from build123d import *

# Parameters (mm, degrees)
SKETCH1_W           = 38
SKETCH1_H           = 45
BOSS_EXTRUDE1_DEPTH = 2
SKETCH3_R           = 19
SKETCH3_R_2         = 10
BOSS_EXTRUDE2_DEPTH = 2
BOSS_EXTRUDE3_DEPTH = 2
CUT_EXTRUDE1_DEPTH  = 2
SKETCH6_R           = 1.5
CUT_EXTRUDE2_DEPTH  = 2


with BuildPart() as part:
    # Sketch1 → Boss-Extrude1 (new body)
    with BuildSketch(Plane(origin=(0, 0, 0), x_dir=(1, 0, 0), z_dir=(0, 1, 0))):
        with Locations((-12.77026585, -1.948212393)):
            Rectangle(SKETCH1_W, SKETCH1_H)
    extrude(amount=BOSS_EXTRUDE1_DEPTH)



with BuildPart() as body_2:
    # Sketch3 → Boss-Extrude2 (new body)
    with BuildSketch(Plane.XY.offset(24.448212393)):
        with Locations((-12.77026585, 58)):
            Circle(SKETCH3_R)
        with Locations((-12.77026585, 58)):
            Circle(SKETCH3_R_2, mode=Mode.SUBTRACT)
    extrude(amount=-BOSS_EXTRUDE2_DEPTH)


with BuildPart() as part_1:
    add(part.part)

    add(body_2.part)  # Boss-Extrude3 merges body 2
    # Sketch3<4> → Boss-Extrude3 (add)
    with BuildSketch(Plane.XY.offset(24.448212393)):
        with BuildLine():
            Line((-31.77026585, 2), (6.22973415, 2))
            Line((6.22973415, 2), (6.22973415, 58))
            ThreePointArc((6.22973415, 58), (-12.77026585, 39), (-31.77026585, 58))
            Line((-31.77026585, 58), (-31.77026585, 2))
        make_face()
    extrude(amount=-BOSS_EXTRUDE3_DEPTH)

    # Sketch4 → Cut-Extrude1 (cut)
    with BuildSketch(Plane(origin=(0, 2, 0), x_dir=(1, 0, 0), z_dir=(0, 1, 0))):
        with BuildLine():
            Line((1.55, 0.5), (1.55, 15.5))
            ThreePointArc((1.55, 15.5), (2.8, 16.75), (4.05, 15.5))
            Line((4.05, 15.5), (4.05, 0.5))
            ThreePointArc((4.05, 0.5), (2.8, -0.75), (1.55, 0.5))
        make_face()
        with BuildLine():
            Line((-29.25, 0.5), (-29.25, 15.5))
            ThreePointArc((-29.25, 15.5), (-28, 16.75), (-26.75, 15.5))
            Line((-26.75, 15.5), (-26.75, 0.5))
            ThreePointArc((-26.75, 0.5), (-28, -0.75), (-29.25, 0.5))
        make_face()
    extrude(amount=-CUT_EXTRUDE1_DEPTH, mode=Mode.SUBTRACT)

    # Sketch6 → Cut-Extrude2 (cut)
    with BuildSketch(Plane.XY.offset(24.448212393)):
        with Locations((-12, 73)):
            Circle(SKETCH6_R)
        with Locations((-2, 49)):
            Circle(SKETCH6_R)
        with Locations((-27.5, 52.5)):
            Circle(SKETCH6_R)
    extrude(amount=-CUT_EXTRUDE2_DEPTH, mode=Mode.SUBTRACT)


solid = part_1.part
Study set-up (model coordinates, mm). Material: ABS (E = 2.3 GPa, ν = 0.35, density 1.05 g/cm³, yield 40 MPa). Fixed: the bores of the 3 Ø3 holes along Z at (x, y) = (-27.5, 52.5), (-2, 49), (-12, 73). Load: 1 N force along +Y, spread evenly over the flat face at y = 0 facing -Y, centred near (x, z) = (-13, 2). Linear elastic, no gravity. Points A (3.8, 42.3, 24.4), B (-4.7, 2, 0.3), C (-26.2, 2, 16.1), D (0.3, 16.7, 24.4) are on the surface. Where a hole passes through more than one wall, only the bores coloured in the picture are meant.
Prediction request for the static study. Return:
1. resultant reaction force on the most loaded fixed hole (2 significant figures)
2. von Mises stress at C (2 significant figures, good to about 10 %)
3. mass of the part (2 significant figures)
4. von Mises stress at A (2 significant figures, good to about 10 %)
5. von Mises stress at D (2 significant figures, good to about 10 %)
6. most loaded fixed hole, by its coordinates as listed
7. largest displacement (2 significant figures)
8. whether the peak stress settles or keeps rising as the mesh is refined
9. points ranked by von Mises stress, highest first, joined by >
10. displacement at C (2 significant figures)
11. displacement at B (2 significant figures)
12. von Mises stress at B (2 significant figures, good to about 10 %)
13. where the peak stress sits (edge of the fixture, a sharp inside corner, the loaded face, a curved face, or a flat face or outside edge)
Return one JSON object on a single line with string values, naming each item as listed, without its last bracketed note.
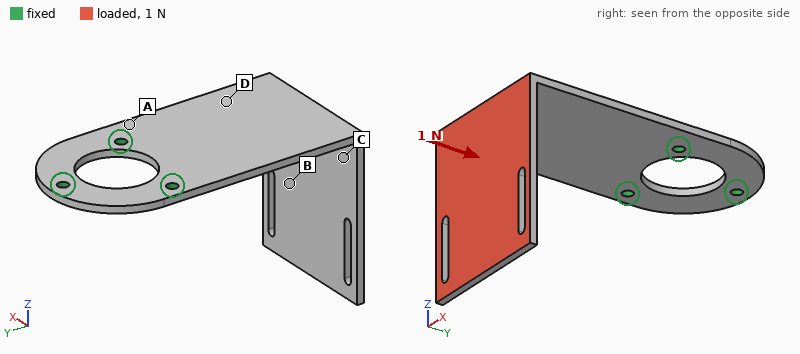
{"resultant reaction force on the most loaded fixed hole": "0.56 N", "von Mises stress at C": "0.50 MPa", "mass of the part": "8.4 g", "von Mises stress at A": "1.00 MPa", "von Mises stress at D": "0.80 MPa", "most loaded fixed hole, by its coordinates as listed": "(-2, 49)", "largest displacement": "1.0 mm", "whether the peak stress settles or keeps rising as the mesh is refined": "keeps rising", "points ranked by von Mises stress, highest first, joined by >": "A > D > C > B", "displacement at C": "0.46 mm", "displacement at B": "0.63 mm", "von Mises stress at B": "0.19 MPa", "where the peak stress sits": "edge of the fixture"}
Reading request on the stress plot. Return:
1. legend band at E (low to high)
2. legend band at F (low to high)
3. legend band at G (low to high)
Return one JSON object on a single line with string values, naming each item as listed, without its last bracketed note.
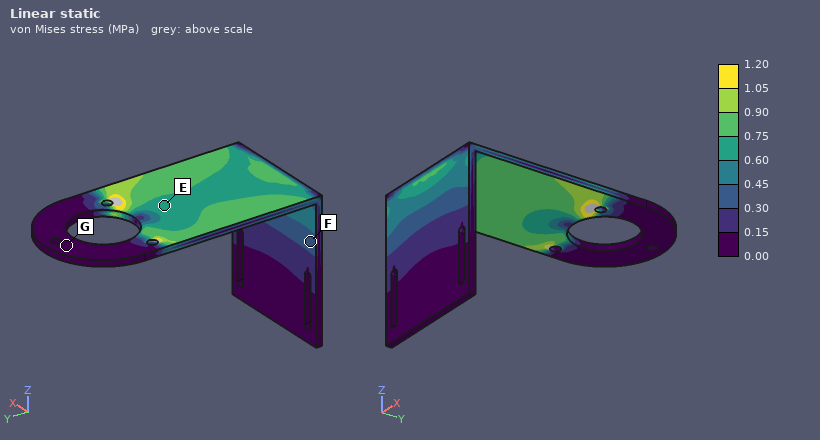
{"legend band at E": "0.60 to 0.75 MPa", "legend band at F": "0.30 to 0.45 MPa", "legend band at G": "0.00 to 0.15 MPa"}
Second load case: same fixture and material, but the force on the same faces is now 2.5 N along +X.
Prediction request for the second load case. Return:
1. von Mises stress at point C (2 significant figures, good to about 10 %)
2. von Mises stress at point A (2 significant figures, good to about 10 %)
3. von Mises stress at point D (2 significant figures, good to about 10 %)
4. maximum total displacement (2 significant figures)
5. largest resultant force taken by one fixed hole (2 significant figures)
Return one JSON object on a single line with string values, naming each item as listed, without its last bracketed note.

{"von Mises stress at point C": "0.68 MPa", "von Mises stress at point A": "1.4 MPa", "von Mises stress at point D": "1.5 MPa", "maximum total displacement": "1.1 mm", "largest resultant force taken by one fixed hole": "4.9 N"}
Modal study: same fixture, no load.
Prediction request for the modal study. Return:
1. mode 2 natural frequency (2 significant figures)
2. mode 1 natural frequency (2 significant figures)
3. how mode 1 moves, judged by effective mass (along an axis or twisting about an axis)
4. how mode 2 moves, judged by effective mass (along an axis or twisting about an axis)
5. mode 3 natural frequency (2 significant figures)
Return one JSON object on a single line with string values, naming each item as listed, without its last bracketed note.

{"mode 2 natural frequency": "150 Hz", "mode 1 natural frequency": "73 Hz", "how mode 1 moves, judged by effective mass": "along Z", "how mode 2 moves, judged by effective mass": "along X", "mode 3 natural frequency": "220 Hz"}
